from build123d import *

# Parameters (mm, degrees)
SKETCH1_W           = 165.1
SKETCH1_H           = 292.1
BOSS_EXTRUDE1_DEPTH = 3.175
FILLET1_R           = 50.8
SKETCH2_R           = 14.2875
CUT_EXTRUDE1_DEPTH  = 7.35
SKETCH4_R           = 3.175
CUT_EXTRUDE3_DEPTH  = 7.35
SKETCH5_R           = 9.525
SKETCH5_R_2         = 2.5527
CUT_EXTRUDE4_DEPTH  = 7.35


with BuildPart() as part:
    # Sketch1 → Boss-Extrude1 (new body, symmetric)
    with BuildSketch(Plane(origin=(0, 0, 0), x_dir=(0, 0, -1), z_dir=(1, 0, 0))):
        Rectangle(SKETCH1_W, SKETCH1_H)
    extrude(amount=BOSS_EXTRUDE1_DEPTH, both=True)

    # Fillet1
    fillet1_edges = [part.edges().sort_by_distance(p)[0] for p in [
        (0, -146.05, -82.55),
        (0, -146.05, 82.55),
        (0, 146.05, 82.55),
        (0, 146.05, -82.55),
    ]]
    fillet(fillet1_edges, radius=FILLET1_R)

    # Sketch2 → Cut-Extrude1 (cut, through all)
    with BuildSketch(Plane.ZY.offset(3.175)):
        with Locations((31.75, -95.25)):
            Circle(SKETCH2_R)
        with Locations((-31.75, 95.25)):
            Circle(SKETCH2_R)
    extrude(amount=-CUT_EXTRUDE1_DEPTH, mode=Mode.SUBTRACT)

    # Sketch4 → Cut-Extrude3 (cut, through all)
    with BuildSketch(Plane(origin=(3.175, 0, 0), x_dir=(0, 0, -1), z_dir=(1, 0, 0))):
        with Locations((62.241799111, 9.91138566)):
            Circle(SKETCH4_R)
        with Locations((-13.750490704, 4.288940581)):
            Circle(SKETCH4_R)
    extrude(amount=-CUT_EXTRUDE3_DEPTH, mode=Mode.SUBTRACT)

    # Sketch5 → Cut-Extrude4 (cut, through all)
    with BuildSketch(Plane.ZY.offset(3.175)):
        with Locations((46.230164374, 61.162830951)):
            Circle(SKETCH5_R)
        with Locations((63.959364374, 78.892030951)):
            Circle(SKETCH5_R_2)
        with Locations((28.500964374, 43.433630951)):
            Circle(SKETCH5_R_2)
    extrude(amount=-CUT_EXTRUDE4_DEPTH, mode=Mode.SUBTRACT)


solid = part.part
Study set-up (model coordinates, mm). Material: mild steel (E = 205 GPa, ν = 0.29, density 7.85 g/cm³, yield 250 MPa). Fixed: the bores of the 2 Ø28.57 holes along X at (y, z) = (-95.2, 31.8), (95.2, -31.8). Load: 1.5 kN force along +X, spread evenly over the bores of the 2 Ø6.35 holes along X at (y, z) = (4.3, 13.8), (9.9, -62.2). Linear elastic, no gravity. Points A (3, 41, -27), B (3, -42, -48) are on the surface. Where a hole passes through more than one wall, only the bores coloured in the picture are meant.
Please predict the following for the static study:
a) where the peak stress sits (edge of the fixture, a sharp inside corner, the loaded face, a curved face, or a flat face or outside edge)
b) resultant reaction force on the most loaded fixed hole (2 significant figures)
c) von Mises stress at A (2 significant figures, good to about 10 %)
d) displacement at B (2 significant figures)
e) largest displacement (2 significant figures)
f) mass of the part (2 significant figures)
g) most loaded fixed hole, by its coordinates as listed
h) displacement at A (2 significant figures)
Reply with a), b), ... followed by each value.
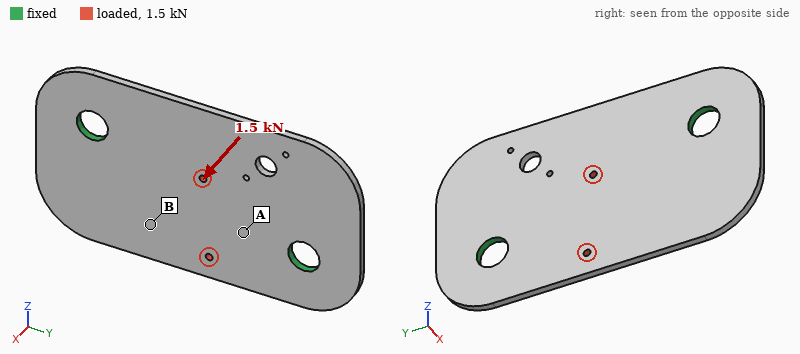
a) the loaded face
b) 900 N
c) 20 MPa
d) 0.11 mm
e) 0.18 mm
f) 2.2 kg
g) (95.2, -31.8)
h) 0.054 mm
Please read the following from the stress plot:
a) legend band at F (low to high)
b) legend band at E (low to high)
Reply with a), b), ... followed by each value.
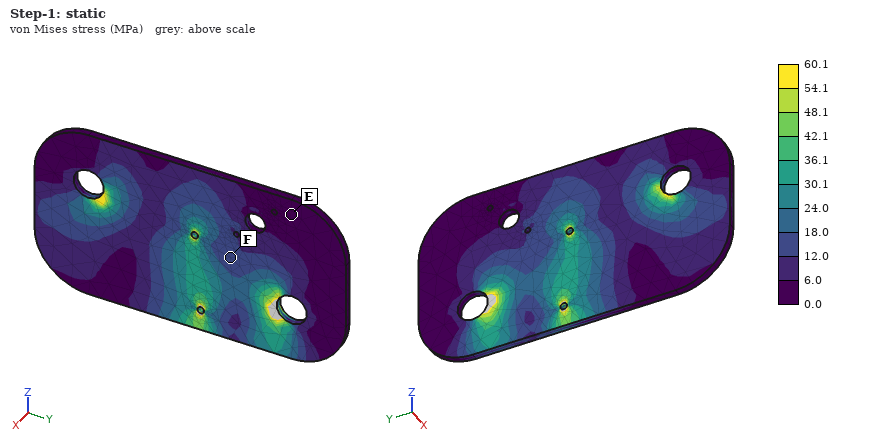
a) 12.0 to 18.0 MPa
b) 0.0 to 6.0 MPa
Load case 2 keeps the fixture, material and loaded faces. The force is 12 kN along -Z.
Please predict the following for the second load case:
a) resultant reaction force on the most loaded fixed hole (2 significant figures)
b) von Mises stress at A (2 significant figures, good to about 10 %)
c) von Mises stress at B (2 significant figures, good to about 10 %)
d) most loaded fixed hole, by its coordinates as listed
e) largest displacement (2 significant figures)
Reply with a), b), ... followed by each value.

a) 6.4 kN
b) 16 MPa
c) 11 MPa
d) (95.2, -31.8)
e) 14 µm
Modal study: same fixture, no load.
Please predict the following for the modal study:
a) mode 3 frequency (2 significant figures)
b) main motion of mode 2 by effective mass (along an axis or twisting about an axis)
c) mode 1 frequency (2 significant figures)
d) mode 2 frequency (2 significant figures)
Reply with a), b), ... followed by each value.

a) 930 Hz
b) along X
c) 520 Hz
d) 600 Hz
